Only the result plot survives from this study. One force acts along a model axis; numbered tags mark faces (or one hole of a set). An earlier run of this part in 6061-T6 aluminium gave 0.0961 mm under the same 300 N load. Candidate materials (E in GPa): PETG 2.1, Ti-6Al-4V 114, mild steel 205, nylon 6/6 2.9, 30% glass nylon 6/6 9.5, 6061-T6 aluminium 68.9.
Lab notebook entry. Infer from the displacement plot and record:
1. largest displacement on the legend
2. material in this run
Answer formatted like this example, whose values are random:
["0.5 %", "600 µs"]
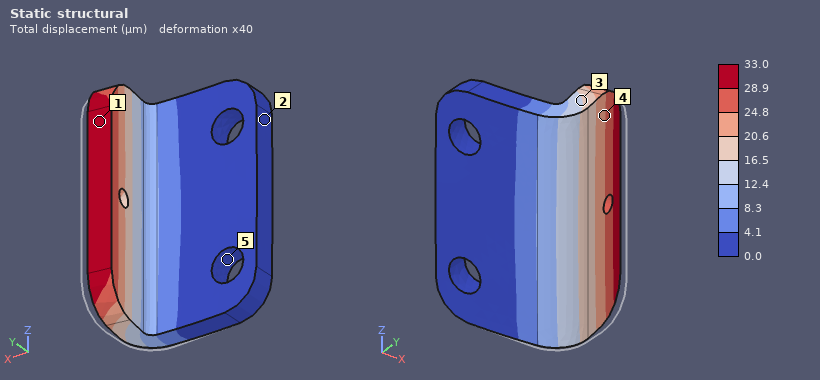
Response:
["33.0 µm", "mild steel"]
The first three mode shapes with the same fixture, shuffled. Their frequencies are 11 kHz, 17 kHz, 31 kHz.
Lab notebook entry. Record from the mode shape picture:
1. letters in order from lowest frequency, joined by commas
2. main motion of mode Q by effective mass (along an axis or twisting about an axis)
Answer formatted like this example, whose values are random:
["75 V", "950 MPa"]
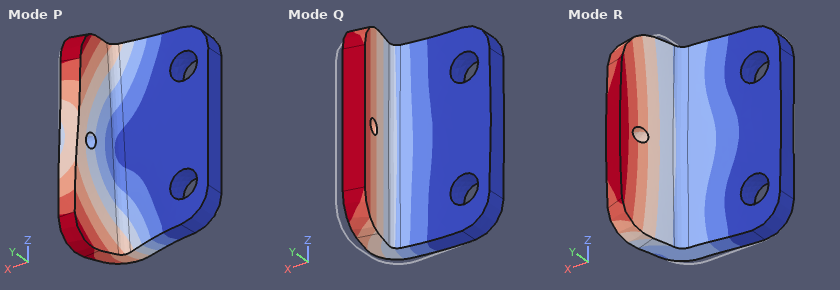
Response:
["Q, P, R", "along Y"]
